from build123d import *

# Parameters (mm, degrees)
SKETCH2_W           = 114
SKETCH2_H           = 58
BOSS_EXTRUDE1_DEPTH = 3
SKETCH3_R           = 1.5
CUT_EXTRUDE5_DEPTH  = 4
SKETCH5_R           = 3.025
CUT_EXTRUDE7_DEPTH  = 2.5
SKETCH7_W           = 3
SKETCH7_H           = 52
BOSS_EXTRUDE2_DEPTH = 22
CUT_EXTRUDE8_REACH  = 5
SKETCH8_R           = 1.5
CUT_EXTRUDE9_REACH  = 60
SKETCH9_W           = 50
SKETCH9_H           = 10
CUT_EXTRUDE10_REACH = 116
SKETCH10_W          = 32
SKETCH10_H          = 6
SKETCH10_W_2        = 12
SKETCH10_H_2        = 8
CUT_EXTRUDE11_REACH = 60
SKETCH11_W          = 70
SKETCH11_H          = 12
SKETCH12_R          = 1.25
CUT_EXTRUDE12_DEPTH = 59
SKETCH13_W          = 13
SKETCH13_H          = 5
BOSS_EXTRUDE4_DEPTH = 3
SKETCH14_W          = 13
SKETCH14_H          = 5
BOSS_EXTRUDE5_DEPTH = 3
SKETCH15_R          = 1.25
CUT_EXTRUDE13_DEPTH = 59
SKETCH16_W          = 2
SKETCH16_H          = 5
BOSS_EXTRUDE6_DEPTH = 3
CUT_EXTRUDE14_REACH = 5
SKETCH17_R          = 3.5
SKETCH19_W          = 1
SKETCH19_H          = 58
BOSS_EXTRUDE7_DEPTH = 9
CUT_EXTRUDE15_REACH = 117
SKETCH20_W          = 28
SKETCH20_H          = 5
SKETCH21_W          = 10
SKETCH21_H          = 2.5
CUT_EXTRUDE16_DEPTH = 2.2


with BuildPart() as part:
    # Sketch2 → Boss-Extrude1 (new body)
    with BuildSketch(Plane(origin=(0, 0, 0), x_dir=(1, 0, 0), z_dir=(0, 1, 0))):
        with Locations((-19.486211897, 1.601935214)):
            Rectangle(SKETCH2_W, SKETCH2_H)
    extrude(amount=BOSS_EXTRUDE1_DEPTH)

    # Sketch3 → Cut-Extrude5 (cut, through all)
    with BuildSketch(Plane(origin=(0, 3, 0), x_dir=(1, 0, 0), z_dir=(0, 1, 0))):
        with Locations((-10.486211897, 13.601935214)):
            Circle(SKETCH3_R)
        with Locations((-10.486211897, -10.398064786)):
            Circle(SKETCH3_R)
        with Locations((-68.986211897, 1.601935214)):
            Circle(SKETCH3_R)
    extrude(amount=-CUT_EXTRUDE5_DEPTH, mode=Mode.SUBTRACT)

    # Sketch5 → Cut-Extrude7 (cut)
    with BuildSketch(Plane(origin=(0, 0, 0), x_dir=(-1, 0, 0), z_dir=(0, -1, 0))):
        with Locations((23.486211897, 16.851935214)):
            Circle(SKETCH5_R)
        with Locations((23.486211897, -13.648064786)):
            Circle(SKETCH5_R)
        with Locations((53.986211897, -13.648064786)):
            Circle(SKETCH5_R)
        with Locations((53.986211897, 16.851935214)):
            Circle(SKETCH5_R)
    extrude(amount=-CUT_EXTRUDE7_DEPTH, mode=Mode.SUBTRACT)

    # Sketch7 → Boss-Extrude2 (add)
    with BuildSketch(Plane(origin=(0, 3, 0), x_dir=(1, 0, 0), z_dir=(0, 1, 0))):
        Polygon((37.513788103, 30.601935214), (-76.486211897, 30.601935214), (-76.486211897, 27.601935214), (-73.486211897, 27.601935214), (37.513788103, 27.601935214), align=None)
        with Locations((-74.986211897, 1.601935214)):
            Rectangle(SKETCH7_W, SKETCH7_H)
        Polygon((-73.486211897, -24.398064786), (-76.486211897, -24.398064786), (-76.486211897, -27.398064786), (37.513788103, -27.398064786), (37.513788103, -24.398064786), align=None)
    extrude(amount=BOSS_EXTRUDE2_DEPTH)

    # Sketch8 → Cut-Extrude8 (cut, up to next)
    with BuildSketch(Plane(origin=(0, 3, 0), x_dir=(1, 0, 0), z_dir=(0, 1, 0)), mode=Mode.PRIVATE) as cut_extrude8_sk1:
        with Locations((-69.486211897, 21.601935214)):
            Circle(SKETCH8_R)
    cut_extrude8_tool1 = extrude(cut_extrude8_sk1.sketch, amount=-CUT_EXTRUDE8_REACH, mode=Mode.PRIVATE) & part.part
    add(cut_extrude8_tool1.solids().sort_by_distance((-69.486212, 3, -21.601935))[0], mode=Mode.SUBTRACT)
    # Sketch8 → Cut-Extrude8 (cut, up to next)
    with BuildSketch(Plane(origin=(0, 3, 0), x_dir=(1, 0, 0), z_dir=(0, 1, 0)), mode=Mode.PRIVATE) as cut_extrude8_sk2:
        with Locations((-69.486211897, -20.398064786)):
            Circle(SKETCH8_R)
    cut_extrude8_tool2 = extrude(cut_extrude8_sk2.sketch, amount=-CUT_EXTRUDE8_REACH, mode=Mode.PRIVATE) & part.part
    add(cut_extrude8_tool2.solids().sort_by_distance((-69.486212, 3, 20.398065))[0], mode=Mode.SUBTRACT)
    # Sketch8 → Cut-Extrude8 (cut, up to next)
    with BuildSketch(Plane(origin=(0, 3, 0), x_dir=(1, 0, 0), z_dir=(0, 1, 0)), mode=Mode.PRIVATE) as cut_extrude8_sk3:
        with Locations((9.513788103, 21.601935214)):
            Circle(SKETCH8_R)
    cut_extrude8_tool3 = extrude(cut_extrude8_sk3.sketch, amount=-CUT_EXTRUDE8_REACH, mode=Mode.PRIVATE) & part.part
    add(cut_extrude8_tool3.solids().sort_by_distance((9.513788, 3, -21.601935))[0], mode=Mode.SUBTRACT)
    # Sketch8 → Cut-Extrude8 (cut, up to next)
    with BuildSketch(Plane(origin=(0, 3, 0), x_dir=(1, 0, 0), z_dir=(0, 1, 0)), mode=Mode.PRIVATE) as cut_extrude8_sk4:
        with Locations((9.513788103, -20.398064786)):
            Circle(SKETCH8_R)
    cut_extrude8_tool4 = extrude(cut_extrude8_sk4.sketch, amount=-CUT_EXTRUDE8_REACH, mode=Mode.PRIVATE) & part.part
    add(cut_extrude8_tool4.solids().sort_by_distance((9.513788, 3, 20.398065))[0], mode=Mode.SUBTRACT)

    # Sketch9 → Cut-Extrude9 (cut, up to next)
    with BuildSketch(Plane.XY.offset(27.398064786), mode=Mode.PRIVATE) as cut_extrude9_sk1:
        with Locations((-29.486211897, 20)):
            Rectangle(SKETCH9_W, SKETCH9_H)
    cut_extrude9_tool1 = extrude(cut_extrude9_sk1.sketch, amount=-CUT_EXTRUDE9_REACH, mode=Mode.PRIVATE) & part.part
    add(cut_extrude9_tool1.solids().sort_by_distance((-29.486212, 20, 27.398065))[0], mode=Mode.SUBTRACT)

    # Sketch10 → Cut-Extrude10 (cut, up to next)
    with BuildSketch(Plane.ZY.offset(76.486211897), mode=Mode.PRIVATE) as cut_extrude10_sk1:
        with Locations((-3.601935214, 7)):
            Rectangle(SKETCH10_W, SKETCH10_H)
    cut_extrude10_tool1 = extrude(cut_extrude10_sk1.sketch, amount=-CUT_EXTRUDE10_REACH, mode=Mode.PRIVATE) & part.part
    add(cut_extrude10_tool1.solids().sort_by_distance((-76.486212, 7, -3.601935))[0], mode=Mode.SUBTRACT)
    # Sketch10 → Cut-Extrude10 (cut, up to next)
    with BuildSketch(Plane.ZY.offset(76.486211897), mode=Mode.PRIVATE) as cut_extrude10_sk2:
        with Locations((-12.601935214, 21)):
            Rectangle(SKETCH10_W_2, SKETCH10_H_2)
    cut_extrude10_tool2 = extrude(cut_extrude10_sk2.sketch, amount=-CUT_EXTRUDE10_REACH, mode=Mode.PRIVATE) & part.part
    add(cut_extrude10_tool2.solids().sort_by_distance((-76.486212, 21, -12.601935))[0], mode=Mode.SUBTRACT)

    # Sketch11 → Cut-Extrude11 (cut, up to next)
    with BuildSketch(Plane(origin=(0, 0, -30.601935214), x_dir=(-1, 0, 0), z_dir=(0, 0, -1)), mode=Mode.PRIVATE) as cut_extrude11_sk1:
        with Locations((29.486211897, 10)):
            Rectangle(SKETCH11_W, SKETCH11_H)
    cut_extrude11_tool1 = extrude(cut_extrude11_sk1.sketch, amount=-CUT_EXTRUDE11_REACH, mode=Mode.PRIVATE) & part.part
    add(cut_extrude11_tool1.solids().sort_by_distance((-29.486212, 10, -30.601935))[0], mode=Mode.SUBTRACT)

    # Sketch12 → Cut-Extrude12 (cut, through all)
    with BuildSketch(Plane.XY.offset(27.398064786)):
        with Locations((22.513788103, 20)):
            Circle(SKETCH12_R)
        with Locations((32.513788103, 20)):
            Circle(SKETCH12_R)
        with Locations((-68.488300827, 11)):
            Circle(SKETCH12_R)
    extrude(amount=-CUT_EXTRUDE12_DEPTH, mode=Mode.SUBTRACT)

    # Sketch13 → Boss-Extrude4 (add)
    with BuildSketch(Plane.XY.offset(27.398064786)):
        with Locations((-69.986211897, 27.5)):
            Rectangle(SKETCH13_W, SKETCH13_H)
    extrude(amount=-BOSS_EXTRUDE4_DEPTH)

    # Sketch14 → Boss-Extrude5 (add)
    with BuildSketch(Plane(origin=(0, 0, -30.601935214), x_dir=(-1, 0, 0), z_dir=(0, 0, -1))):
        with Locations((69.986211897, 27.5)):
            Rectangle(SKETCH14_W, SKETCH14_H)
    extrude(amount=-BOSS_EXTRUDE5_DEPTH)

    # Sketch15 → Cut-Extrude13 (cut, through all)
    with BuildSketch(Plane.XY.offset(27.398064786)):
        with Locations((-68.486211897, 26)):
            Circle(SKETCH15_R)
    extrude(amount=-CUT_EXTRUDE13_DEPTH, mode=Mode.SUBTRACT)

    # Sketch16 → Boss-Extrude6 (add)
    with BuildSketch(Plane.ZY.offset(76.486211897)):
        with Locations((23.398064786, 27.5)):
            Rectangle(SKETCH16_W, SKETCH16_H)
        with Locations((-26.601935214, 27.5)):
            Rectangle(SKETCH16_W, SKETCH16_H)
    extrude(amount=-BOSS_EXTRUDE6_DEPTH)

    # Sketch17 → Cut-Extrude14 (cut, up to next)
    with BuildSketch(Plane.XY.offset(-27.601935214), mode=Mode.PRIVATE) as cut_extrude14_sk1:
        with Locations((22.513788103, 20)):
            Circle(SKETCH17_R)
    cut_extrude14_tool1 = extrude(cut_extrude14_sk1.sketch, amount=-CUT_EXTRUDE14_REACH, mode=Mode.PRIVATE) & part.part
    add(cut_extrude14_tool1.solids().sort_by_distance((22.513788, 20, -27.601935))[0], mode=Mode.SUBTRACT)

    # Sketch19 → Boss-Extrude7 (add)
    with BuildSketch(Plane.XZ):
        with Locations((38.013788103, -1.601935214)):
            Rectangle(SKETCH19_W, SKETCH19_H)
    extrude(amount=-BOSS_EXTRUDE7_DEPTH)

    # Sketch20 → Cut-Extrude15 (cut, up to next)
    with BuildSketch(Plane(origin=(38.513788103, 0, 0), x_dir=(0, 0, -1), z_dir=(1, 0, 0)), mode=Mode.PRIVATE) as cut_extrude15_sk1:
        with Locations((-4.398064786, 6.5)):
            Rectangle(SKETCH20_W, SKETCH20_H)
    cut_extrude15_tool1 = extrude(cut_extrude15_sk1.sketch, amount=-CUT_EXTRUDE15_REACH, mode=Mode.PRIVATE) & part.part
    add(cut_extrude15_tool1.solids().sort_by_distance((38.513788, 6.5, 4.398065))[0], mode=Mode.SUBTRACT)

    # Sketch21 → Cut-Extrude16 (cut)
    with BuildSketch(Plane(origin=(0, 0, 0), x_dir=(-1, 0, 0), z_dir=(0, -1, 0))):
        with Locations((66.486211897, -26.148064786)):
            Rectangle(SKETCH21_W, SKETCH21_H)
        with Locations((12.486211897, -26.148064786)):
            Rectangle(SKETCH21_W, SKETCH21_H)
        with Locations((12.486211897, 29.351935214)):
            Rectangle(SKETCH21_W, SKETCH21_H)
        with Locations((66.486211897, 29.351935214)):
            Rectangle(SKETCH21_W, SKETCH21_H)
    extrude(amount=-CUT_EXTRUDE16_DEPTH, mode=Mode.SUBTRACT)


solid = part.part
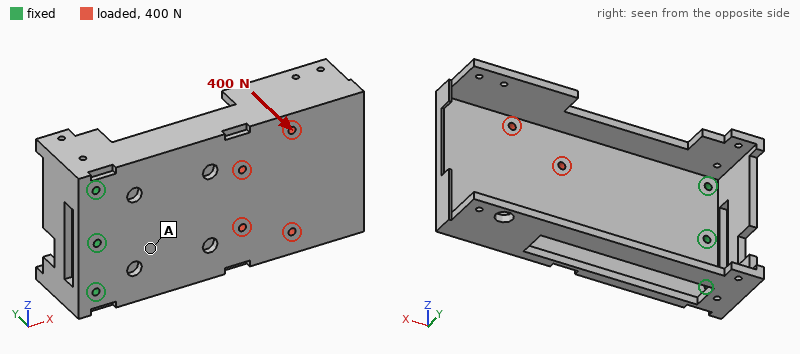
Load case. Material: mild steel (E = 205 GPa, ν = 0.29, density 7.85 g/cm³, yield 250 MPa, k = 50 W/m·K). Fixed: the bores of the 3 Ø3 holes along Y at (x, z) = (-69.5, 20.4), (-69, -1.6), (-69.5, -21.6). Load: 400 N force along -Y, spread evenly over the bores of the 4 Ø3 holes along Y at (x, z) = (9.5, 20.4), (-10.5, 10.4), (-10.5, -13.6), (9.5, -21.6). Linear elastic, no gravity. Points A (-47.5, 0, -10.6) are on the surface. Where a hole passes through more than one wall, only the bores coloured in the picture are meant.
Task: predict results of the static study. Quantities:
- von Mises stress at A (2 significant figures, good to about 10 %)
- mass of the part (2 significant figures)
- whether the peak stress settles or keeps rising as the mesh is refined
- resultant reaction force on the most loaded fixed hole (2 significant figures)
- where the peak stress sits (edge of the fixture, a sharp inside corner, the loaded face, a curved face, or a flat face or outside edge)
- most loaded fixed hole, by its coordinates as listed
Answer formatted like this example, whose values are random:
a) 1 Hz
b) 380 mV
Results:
a) 38 MPa
b) 260 g
c) keeps rising
d) 510 N
e) edge of the fixture
f) (-69, -1.6)
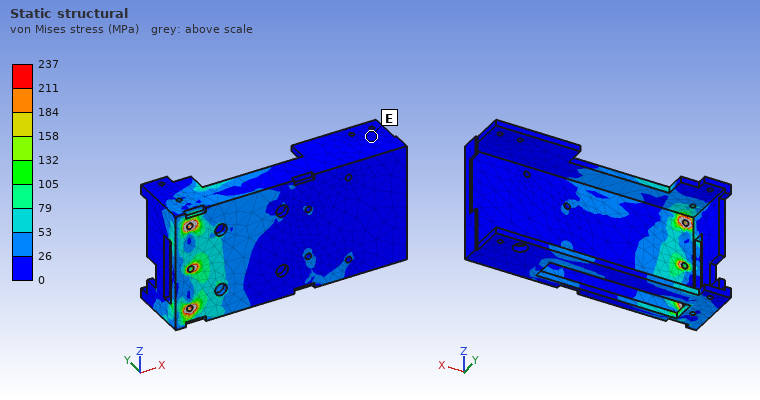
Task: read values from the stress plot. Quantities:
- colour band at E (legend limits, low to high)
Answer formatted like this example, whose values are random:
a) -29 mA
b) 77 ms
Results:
a) 0 to 26 MPa
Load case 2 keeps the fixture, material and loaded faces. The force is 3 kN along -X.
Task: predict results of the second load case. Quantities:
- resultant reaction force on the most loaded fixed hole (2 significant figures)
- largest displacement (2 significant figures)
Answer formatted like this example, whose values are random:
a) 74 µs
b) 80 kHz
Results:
a) 1.0 kN
b) 34 µm
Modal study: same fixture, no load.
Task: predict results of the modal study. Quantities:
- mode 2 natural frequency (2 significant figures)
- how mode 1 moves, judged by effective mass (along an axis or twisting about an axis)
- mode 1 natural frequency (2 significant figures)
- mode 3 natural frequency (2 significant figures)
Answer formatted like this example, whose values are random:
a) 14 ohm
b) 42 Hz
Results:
a) 680 Hz
b) along Y
c) 380 Hz
d) 1700 Hz
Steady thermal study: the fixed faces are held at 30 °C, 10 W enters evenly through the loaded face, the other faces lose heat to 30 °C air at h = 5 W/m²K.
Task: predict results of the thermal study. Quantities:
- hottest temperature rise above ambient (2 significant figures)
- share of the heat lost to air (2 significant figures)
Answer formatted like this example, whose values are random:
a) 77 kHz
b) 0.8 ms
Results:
a) 49 K
b) 34 %
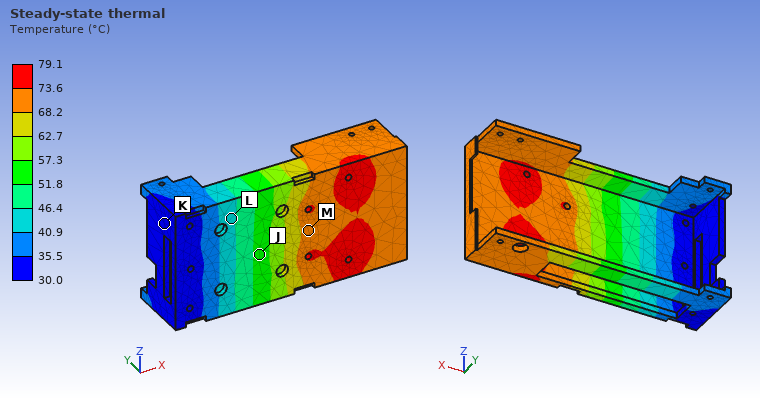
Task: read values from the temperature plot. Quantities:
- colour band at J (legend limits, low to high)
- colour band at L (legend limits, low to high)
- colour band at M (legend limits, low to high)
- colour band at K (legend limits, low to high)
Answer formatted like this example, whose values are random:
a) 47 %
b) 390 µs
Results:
a) 51.8 to 57.3 °C
b) 40.9 to 46.4 °C
c) 68.2 to 73.6 °C
d) 30.0 to 35.5 °C
